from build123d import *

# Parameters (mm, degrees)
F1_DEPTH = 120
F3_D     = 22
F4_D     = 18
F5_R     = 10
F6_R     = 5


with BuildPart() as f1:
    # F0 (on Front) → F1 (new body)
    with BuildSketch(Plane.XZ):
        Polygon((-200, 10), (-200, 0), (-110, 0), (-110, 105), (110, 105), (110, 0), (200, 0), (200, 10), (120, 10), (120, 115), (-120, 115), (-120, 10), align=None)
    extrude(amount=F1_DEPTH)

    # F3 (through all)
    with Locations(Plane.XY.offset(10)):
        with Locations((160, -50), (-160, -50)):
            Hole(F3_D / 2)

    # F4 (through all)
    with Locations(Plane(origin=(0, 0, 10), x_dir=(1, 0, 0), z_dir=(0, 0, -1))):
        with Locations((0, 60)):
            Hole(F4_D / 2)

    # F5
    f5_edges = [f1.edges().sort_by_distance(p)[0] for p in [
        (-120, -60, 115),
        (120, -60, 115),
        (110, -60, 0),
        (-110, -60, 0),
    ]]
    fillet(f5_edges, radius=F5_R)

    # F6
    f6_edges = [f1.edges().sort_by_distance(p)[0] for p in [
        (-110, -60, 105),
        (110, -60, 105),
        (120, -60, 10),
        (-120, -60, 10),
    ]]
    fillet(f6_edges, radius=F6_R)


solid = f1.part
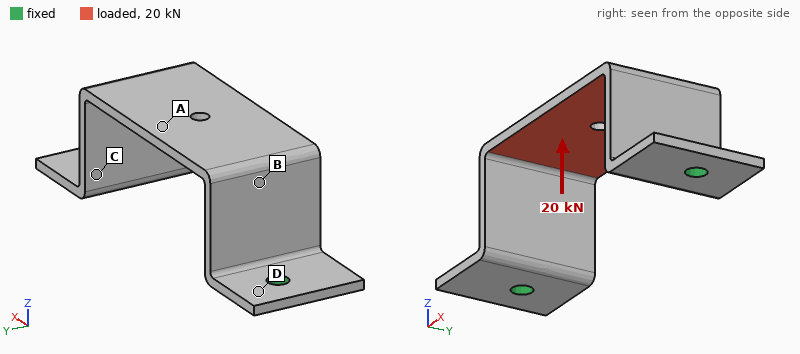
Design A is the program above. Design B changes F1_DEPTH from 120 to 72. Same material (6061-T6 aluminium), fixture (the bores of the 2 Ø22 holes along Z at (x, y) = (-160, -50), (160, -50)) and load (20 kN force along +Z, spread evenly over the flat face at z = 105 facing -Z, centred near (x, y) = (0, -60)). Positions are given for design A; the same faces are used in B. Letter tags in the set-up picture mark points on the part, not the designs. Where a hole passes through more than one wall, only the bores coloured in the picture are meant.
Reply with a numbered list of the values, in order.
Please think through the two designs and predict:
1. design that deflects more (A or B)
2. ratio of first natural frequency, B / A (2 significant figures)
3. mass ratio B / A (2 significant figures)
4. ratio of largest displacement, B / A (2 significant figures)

1. B
2. 1.0
3. 0.59
4. 1.6
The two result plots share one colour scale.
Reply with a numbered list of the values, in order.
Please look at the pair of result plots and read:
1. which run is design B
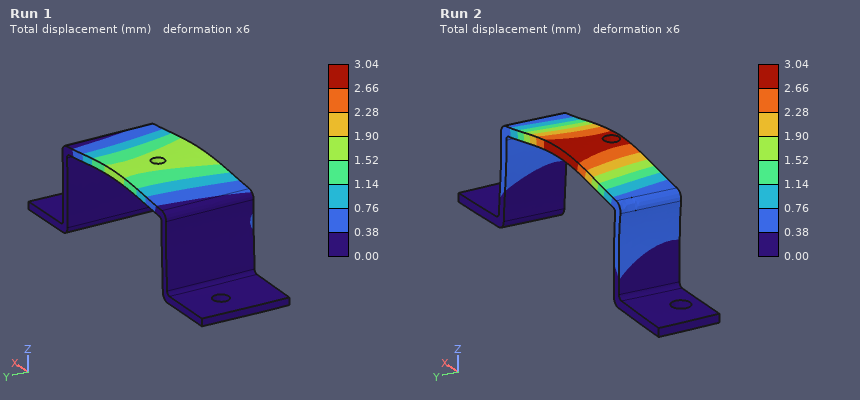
1. Run 2
